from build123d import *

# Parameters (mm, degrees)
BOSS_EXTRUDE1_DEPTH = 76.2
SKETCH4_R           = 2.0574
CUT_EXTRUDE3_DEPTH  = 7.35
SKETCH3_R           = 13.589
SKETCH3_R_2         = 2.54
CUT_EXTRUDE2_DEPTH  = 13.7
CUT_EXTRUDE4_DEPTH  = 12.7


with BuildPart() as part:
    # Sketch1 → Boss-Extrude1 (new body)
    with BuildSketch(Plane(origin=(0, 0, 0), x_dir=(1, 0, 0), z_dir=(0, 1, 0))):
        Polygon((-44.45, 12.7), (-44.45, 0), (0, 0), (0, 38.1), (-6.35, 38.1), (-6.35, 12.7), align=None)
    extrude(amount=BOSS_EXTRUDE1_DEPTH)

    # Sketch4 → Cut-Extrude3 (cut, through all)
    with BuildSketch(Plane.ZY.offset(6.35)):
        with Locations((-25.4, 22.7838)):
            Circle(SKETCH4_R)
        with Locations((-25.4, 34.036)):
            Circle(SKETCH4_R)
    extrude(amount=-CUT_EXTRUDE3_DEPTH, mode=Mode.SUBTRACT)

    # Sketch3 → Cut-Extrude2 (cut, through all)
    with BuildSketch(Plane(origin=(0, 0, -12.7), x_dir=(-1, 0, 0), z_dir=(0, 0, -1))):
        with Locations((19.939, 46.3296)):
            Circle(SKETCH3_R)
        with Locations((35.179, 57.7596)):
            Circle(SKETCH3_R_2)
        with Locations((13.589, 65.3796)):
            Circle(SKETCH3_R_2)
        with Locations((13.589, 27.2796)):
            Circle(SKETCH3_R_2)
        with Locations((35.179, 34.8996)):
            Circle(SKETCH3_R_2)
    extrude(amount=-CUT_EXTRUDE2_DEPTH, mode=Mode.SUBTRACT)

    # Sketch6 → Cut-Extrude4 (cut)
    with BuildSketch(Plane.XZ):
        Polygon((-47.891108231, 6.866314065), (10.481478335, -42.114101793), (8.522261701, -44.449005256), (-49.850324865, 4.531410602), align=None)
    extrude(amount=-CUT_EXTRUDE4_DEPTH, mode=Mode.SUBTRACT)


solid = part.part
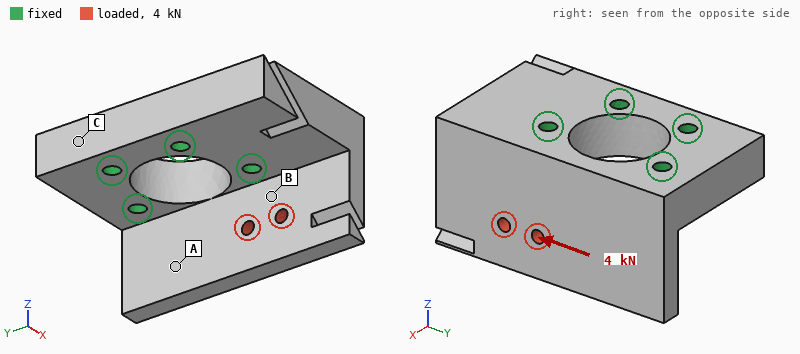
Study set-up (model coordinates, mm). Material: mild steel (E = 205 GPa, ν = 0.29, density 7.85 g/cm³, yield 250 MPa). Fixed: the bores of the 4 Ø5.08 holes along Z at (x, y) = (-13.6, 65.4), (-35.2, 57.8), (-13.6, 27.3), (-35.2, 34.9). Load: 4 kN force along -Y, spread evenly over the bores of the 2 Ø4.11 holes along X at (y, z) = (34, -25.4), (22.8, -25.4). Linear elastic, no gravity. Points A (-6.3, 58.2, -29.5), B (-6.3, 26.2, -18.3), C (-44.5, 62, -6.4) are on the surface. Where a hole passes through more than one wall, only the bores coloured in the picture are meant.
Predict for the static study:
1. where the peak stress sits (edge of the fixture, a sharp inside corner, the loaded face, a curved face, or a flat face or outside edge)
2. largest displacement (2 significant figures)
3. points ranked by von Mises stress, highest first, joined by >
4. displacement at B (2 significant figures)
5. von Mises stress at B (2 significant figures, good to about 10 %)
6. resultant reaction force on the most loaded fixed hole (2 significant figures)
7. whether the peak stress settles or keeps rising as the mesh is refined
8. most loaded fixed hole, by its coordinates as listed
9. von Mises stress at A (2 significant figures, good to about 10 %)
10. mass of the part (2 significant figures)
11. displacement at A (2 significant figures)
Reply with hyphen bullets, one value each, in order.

- edge of the fixture
- 10 µm
- B > A > C
- 4.1 µm
- 28 MPa
- 3.3 kN
- keeps rising
- (-13.6, 27.3)
- 13 MPa
- 360 g
- 5.1 µm
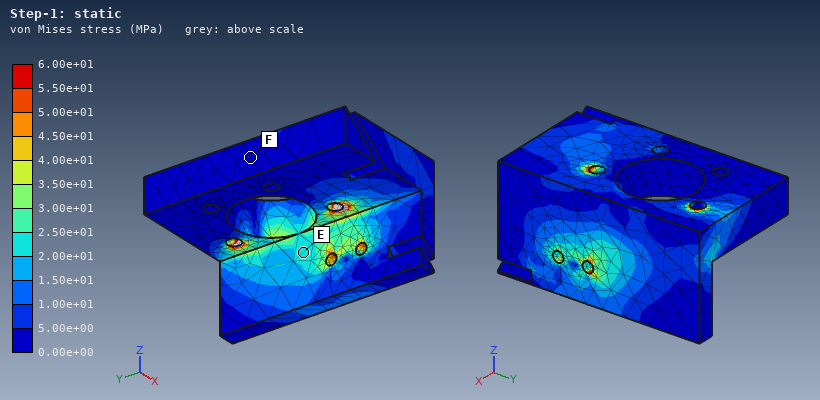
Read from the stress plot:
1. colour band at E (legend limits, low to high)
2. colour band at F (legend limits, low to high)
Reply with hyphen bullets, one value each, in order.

- 2.00e+01 to 2.50e+01 MPa
- 0.00e+00 to 5.00e+00 MPa
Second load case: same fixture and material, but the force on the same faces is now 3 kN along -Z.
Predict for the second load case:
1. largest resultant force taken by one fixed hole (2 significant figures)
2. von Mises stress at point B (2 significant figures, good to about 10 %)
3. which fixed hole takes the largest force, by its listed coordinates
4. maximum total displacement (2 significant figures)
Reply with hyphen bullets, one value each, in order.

- 2.9 kN
- 22 MPa
- (-13.6, 27.3)
- 8.4 µm
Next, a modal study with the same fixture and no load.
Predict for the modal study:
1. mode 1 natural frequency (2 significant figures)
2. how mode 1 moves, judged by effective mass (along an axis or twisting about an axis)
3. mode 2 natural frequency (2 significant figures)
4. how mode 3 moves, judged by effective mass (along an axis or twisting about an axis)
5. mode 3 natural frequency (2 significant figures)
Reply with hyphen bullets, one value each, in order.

- 5400 Hz
- along X
- 7300 Hz
- along Z
- 10 kHz
